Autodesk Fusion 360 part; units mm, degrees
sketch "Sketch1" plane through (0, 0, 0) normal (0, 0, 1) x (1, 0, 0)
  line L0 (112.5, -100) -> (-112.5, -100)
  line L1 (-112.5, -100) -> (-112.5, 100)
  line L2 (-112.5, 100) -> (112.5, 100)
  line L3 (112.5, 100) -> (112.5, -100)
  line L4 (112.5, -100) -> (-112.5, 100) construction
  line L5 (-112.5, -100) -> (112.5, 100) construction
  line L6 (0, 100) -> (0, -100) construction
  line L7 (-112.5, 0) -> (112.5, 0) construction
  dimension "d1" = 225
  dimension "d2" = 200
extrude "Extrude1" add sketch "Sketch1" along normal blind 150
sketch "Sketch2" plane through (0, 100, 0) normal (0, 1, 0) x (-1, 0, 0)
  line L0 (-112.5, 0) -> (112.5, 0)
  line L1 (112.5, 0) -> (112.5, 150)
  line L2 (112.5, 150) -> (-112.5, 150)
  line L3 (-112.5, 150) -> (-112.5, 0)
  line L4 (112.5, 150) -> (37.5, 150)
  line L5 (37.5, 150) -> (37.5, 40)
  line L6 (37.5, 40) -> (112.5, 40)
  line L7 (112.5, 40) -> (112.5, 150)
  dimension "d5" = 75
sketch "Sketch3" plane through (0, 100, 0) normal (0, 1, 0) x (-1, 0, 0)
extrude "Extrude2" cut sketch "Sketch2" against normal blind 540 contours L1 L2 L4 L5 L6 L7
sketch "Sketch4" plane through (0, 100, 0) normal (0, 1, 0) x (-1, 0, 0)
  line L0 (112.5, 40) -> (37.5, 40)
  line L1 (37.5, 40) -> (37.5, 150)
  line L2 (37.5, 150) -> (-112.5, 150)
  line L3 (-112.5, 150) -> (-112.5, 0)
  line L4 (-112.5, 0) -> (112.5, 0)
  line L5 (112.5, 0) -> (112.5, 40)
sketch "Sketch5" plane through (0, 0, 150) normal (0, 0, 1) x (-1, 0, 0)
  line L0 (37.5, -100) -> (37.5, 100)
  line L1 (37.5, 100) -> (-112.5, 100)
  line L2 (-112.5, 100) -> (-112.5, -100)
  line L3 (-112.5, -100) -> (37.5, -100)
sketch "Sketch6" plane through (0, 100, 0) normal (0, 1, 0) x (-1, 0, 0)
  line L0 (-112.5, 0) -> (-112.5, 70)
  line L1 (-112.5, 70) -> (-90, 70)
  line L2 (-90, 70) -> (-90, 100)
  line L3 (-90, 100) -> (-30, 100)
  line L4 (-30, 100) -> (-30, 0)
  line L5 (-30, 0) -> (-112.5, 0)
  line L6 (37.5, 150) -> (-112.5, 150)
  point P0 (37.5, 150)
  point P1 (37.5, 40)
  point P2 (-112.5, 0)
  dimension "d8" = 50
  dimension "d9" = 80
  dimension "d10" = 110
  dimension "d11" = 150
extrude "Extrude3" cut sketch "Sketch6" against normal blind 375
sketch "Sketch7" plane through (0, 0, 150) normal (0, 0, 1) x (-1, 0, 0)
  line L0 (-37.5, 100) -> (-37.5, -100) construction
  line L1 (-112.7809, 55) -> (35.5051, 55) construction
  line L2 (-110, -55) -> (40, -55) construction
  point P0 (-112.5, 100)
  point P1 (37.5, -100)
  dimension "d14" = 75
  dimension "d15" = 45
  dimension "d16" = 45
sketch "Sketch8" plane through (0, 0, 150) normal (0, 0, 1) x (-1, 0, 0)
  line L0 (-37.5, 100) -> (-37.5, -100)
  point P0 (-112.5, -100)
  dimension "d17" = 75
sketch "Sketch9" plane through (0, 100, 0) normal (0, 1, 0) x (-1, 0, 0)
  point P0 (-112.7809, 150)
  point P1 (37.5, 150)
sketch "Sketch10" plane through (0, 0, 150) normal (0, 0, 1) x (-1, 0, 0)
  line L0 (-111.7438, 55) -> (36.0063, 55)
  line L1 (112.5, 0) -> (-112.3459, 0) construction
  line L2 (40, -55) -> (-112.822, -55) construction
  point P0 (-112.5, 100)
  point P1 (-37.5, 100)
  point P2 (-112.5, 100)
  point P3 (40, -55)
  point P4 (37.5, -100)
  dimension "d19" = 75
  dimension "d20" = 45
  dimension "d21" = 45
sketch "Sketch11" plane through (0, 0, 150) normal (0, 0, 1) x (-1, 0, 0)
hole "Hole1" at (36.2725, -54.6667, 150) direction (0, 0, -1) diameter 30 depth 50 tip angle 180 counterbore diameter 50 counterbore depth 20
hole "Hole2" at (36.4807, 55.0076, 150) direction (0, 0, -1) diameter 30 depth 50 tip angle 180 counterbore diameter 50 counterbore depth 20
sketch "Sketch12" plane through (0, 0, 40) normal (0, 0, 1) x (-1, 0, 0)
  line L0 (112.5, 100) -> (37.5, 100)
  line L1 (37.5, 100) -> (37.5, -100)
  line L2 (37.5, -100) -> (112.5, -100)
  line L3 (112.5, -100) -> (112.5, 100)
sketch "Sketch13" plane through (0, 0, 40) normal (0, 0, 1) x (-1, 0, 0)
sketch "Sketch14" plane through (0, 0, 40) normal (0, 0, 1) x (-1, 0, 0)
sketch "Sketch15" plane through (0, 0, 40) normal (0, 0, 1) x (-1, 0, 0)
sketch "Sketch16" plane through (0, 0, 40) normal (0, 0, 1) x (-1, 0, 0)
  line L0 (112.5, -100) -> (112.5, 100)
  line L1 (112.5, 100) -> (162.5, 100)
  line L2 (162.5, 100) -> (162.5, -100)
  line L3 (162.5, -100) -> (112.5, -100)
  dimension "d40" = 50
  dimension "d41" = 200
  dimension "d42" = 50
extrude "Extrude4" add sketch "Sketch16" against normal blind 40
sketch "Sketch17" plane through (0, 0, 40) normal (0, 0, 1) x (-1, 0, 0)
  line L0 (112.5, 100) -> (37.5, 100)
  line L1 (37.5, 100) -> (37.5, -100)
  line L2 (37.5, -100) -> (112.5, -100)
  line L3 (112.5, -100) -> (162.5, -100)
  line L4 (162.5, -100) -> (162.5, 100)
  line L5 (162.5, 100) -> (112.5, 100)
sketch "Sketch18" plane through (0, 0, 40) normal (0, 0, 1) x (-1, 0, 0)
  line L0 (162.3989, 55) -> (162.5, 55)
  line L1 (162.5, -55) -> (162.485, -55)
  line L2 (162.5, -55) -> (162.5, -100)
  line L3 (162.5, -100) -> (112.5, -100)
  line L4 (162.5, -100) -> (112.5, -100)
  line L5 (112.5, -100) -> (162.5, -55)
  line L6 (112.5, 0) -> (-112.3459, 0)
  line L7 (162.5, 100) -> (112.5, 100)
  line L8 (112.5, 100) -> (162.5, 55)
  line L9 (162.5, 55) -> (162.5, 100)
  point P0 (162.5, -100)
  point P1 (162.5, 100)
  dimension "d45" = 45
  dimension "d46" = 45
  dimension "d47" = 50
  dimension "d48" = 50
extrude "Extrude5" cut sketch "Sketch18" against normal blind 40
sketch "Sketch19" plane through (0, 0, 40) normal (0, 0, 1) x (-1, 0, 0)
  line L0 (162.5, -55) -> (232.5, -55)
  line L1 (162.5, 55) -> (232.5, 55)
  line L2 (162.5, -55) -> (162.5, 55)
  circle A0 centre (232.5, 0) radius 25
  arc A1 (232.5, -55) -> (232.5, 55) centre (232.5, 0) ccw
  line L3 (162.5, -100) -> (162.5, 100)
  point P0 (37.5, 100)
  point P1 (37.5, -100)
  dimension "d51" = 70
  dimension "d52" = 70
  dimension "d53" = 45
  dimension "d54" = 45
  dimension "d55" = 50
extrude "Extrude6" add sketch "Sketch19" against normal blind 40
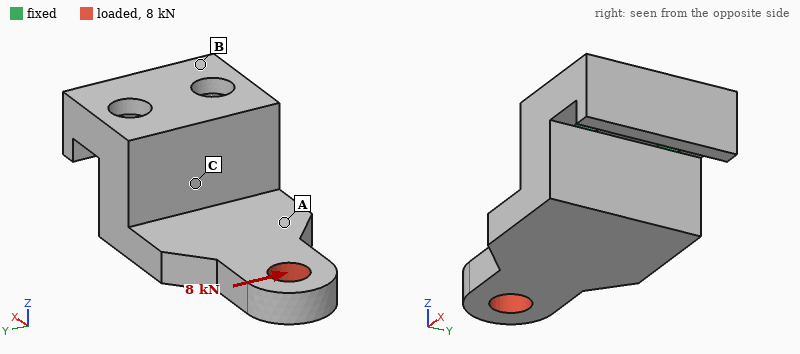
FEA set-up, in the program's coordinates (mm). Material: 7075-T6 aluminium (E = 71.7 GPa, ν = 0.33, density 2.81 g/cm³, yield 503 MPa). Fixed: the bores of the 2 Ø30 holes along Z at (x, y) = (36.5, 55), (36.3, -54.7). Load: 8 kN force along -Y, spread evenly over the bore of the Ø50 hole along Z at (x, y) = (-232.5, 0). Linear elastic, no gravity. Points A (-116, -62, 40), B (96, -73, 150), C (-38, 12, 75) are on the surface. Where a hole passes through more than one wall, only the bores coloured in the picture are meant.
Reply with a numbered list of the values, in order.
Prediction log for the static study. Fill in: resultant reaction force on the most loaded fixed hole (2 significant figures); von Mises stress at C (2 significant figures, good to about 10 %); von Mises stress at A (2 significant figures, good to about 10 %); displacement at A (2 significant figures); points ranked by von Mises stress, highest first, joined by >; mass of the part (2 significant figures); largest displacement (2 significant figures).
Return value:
1. 19 kN
2. 9.7 MPa
3. 5.4 MPa
4. 0.053 mm
5. C > A > B
6. 12 kg
7. 0.14 mm
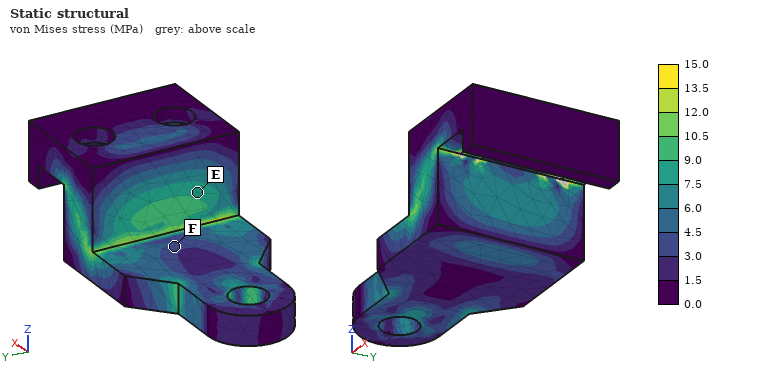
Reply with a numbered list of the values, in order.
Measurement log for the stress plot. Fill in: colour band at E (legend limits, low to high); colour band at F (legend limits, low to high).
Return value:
1. 7.5 to 9.0 MPa
2. 3.0 to 4.5 MPa
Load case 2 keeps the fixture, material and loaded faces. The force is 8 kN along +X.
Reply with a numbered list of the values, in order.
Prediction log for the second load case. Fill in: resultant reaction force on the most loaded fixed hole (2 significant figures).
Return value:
1. 4.1 kN
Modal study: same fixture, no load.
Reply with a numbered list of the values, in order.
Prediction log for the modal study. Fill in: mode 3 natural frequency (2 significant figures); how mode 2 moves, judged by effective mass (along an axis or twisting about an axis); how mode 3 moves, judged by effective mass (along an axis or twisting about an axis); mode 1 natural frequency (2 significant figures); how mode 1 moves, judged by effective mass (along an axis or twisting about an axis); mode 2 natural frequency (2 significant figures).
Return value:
1. 1200 Hz
2. along Y
3. along X
4. 440 Hz
5. along Z
6. 1100 Hz
